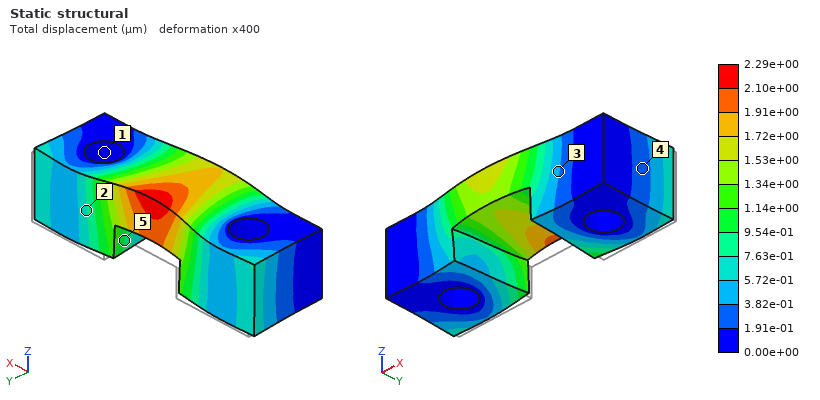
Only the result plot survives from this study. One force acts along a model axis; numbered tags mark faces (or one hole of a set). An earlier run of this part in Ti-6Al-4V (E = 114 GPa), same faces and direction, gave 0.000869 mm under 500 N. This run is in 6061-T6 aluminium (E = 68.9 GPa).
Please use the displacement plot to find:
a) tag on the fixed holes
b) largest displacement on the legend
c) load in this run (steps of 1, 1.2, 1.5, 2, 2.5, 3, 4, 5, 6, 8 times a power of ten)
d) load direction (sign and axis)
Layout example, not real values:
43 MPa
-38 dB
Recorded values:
1
2.29e+00 µm
800 N
-Y
